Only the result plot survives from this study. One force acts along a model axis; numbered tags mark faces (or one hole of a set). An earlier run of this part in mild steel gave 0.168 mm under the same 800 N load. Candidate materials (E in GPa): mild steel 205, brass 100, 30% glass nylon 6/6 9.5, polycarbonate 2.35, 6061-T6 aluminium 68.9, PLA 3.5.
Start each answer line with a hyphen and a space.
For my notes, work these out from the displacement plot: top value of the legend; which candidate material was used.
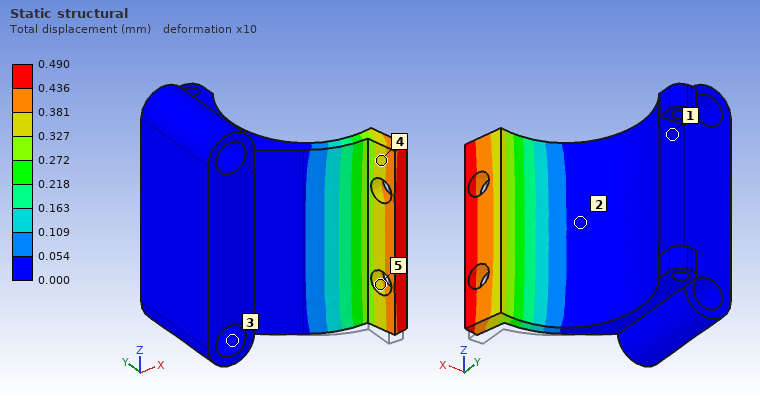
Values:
- 0.490 mm
- 6061-T6 aluminium
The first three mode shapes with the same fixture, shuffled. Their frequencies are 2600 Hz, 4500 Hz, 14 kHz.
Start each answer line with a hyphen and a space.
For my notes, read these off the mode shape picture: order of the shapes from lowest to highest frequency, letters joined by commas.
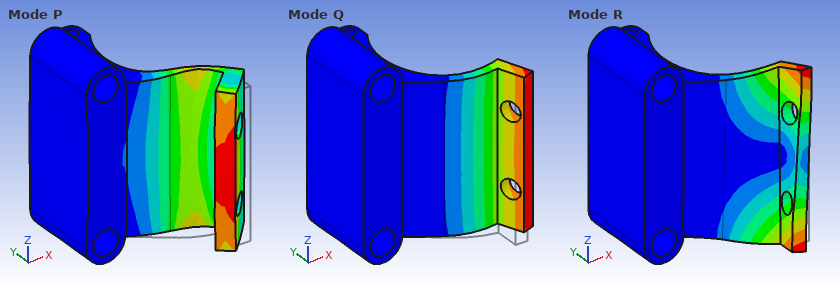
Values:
- Q, R, P
